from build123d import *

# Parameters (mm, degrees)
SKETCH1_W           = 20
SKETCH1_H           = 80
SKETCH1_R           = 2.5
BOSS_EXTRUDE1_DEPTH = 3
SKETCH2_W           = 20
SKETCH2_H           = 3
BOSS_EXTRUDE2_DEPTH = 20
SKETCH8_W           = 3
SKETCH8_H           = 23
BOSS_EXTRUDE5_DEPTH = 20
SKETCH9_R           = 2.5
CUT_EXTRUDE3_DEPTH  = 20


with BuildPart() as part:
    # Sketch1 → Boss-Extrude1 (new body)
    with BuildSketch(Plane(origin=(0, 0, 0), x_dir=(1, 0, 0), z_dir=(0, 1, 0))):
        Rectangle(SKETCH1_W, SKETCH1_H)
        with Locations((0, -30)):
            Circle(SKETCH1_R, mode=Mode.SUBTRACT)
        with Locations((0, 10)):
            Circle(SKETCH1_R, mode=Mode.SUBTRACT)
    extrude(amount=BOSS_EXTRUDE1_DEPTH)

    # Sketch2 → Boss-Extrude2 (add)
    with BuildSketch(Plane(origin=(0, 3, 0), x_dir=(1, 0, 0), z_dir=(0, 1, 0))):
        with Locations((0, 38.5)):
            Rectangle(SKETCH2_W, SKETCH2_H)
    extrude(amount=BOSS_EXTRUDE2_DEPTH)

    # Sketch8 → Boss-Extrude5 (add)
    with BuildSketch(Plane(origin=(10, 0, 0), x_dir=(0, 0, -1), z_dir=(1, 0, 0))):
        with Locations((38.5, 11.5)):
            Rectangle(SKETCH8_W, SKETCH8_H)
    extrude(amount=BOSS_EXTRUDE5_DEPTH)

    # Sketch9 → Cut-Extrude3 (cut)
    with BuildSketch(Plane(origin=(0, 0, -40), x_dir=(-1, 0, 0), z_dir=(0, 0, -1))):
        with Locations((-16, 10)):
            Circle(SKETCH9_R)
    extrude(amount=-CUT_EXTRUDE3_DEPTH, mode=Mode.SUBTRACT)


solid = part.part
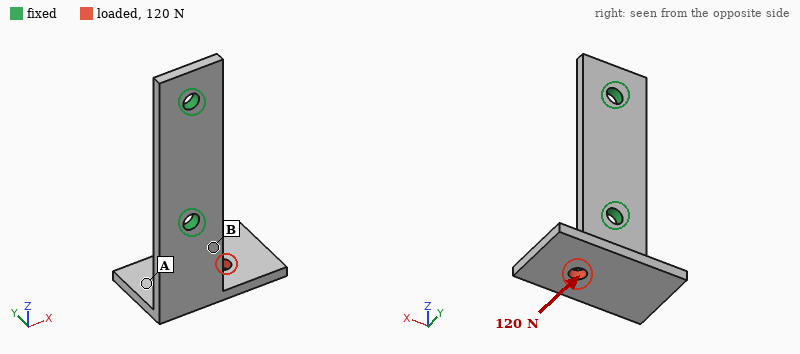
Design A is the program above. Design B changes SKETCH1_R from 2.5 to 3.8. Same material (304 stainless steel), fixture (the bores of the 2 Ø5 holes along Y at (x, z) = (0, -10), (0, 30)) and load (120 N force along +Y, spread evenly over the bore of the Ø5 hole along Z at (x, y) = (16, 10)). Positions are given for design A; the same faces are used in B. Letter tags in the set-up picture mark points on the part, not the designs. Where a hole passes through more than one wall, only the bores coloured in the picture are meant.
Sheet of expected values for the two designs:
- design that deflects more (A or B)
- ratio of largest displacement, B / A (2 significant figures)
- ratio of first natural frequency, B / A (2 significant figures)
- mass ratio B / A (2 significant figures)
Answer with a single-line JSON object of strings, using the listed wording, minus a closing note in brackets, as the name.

{"design that deflects more": "A", "ratio of largest displacement, B / A": "0.88", "ratio of first natural frequency, B / A": "1.1", "mass ratio B / A": "0.98"}
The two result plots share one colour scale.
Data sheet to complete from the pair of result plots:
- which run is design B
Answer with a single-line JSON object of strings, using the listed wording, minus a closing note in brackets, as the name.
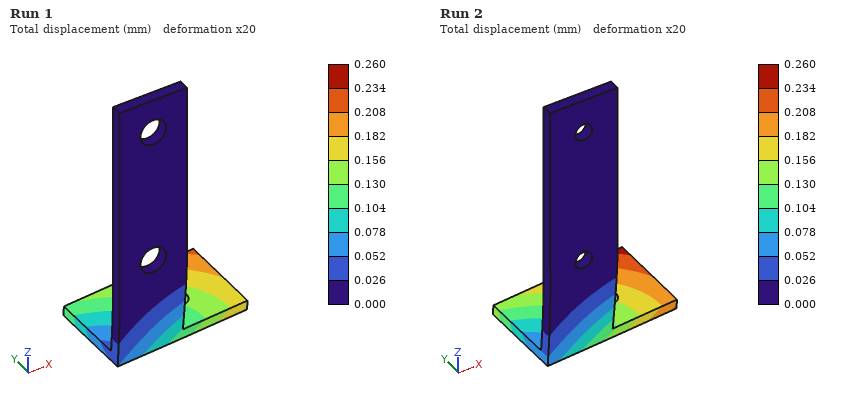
{"which run is design B": "Run 1"}
